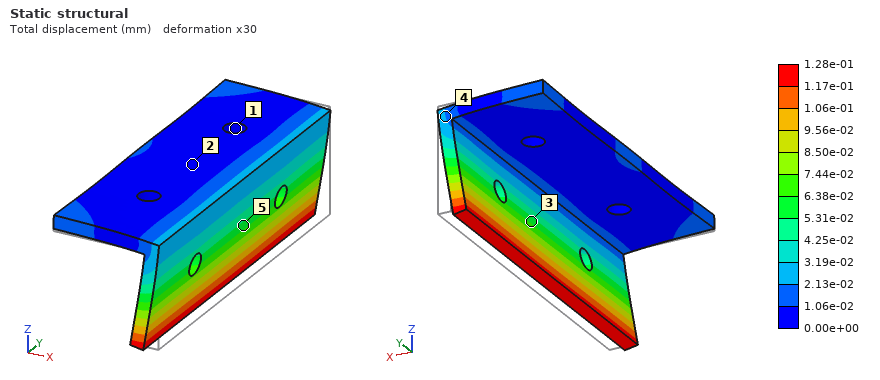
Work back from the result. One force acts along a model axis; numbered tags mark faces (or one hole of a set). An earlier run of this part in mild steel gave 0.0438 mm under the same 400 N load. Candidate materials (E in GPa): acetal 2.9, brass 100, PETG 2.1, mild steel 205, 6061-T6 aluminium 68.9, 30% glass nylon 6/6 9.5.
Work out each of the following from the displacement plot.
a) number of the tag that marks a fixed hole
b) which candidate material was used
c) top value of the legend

1
6061-T6 aluminium
1.28e-01 mm
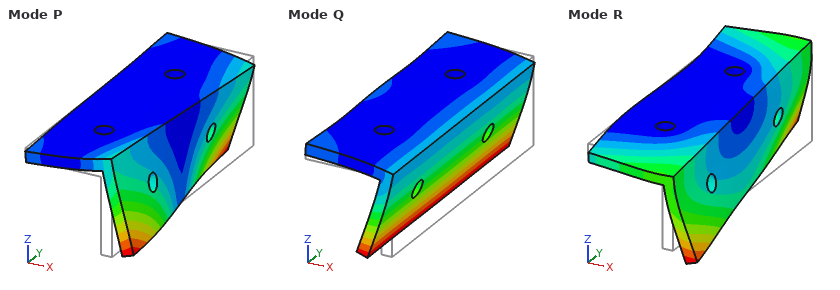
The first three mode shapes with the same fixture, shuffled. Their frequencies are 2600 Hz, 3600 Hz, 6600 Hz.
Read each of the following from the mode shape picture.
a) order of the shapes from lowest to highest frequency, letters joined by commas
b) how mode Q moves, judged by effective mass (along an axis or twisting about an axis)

Q, P, R
along X
